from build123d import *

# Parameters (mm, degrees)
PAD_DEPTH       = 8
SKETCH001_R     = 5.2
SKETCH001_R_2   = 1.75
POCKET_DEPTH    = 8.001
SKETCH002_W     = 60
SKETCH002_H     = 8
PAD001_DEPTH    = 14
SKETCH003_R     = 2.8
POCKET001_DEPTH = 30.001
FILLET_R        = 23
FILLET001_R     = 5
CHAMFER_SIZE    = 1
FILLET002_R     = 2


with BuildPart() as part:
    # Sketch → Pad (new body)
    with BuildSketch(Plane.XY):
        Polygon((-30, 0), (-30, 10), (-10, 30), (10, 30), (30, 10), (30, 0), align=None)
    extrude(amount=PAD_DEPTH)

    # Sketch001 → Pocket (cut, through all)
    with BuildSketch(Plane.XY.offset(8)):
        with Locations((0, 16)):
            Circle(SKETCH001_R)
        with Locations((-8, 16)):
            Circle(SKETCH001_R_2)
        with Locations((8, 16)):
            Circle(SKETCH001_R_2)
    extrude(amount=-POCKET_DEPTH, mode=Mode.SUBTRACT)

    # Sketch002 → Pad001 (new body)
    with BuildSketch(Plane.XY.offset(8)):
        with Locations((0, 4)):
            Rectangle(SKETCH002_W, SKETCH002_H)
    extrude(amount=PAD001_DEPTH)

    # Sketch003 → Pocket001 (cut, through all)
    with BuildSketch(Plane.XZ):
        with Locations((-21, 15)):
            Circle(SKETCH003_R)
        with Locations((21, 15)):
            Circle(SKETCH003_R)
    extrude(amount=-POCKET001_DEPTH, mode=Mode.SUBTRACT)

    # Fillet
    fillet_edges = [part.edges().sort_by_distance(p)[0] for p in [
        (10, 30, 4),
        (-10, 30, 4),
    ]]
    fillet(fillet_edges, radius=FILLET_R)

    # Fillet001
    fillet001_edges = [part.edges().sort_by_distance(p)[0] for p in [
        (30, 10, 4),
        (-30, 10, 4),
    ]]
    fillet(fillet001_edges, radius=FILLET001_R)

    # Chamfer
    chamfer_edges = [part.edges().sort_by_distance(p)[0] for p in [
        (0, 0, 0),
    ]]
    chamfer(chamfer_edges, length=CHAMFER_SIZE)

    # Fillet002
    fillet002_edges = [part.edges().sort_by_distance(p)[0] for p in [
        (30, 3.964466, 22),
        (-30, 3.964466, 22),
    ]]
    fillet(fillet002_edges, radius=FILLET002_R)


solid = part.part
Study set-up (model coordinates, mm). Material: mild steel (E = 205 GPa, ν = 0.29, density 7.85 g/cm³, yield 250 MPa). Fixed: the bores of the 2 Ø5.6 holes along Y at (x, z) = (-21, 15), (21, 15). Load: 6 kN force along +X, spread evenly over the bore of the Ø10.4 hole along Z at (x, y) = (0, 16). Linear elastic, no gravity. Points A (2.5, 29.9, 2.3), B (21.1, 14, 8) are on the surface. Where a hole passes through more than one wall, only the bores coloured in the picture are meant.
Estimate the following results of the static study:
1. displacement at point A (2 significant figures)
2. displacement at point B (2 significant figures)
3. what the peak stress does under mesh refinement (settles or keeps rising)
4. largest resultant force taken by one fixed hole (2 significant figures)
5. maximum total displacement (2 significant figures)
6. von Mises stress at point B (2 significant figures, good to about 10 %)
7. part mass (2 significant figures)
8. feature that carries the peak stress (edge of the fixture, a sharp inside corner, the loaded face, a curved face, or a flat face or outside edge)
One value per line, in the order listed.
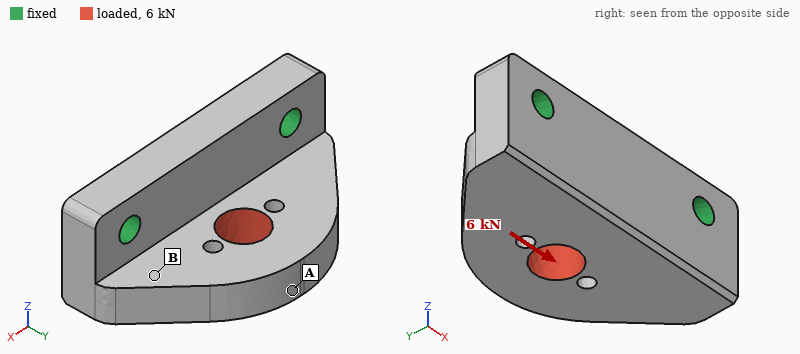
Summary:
8.5 µm
5.8 µm
keeps rising
3.6 kN
10 µm
30 MPa
130 g
edge of the fixture
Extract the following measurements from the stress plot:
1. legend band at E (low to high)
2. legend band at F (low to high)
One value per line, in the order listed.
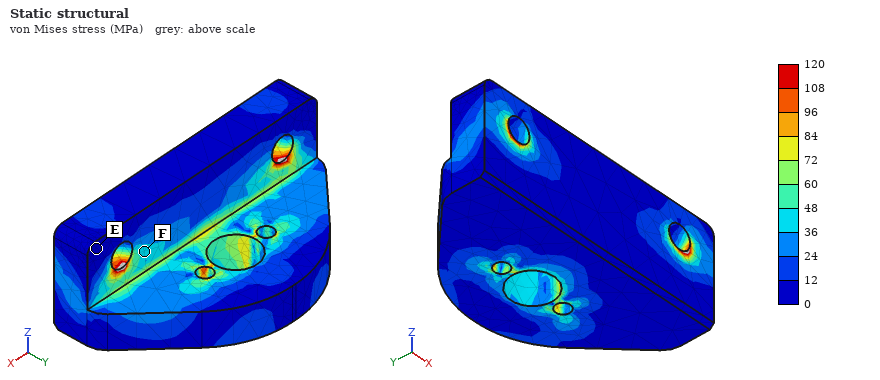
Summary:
0 to 12 MPa
36 to 48 MPa
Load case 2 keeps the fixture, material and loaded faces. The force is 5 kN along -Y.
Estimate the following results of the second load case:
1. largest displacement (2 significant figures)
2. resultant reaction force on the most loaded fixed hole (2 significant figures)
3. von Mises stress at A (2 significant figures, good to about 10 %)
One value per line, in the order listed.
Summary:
28 µm
2.5 kN
30 MPa
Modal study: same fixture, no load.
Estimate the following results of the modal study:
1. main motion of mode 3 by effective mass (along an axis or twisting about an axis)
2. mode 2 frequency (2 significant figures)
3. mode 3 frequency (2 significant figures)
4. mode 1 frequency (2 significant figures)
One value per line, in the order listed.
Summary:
along Y
15 kHz
17 kHz
7200 Hz
